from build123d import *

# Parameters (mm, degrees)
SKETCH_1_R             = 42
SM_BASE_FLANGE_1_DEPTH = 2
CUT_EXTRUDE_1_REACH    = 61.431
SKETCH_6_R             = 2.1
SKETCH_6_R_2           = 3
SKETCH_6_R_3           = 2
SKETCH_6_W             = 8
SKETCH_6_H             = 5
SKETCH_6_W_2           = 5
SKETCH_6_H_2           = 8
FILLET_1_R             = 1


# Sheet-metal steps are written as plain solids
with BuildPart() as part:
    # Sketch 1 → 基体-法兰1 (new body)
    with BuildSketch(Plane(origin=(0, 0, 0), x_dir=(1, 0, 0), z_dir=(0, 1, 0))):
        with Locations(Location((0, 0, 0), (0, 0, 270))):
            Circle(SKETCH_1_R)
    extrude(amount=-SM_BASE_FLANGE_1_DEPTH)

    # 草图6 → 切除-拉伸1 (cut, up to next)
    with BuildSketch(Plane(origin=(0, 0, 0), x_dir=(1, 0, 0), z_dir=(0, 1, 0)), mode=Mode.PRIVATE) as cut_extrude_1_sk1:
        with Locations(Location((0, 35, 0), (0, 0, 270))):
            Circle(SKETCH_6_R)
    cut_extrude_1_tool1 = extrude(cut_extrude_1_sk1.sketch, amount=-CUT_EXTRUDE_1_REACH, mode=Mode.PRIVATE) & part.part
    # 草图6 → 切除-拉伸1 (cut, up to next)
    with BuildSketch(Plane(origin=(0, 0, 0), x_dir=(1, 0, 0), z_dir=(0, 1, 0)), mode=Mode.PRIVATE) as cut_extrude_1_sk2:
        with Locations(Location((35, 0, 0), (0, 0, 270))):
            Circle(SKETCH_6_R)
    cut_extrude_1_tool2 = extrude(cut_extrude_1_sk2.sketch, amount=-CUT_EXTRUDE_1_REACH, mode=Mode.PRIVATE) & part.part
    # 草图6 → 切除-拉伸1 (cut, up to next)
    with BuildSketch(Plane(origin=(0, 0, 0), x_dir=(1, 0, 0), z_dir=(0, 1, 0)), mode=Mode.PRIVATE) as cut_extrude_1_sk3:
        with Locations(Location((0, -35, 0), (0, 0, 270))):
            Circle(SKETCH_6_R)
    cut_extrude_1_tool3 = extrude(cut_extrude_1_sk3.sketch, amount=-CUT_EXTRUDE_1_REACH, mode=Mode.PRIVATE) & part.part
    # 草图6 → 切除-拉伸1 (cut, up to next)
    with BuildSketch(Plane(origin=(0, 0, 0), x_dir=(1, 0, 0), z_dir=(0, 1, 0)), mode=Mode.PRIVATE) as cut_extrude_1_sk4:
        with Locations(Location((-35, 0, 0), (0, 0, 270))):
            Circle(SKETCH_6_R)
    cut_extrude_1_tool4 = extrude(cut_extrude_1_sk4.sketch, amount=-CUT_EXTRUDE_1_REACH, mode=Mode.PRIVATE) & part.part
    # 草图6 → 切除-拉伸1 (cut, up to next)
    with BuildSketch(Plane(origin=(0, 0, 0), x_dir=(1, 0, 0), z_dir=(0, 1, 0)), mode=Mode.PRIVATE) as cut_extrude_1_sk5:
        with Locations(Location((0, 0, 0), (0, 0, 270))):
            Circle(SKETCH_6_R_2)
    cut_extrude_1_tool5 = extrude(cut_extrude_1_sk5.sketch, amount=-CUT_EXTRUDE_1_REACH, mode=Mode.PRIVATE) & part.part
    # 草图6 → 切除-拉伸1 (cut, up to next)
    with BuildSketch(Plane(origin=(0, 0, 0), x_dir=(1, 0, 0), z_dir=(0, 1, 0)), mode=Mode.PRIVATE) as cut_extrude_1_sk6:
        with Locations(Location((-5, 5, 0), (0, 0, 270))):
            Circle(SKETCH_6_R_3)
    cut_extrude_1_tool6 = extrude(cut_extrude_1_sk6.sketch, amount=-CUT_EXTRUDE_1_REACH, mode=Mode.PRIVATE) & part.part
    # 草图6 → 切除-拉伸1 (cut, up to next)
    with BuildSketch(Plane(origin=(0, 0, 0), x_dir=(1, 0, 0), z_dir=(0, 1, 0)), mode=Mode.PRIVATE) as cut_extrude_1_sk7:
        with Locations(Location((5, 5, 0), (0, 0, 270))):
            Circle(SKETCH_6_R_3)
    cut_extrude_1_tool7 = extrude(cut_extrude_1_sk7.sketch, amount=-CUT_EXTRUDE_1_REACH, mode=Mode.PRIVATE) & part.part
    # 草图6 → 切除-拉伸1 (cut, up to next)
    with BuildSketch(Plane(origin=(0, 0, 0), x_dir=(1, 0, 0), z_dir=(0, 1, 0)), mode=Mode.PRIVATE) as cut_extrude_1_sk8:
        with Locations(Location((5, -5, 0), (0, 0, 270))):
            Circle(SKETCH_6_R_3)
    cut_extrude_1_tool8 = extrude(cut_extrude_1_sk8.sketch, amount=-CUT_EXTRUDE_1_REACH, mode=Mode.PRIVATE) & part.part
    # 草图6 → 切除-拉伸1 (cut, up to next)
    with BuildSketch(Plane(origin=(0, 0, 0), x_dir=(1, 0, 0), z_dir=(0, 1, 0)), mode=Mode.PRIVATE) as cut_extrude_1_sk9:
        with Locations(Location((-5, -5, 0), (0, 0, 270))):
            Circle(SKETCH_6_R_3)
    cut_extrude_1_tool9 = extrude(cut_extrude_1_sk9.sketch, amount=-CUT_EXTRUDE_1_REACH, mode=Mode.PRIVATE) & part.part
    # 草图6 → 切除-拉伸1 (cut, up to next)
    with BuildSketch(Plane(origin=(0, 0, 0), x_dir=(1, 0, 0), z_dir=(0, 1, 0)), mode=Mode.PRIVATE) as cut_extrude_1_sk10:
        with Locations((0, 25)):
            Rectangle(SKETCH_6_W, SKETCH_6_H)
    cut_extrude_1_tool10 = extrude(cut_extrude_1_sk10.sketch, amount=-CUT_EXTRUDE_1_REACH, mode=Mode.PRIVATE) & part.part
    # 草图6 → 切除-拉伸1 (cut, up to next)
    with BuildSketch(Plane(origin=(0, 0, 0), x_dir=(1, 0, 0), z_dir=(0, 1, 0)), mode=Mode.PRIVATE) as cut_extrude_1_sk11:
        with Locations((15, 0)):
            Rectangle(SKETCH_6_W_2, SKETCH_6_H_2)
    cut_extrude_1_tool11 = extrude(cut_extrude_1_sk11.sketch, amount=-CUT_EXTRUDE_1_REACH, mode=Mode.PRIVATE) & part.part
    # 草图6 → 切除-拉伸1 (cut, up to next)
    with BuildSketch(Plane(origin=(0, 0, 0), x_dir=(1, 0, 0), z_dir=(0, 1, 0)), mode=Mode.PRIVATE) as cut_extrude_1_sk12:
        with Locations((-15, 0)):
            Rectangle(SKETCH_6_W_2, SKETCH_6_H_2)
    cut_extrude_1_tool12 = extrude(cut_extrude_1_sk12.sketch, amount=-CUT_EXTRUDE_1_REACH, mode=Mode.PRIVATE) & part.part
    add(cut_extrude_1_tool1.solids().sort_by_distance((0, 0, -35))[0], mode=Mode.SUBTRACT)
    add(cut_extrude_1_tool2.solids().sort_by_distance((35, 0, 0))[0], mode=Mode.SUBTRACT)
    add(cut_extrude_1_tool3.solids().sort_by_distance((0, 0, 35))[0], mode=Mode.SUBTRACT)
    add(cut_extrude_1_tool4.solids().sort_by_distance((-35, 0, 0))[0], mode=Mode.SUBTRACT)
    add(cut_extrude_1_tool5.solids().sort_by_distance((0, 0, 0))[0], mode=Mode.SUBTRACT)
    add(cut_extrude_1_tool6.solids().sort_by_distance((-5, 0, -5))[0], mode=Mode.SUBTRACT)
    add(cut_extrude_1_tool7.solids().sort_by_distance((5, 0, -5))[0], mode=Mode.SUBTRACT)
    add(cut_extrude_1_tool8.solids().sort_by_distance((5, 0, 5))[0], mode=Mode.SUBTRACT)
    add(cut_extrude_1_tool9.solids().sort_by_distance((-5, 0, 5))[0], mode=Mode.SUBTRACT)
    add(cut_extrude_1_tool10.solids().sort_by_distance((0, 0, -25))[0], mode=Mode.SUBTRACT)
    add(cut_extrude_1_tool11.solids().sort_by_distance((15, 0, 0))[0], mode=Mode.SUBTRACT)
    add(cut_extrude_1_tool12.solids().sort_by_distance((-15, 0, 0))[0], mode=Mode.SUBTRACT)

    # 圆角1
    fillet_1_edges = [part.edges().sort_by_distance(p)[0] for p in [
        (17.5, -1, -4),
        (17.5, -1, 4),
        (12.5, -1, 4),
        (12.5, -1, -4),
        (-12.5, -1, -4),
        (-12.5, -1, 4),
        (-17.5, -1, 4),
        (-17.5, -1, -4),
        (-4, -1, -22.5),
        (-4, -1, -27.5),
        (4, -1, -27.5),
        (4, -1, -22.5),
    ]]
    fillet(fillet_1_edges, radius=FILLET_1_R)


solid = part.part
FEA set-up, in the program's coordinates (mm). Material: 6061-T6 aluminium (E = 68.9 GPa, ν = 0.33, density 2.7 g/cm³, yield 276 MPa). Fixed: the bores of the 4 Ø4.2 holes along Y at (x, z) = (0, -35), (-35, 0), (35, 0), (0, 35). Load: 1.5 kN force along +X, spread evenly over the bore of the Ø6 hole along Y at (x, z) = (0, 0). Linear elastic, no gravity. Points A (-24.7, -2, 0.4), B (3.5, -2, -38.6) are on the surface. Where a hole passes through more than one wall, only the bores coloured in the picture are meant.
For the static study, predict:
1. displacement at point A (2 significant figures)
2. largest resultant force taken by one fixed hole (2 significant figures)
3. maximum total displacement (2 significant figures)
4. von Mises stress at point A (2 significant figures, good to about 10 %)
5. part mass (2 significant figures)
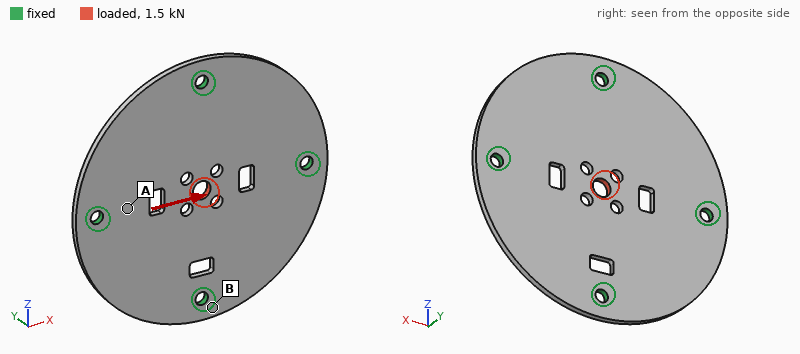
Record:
2.2 µm
460 N
14 µm
13 MPa
29 g
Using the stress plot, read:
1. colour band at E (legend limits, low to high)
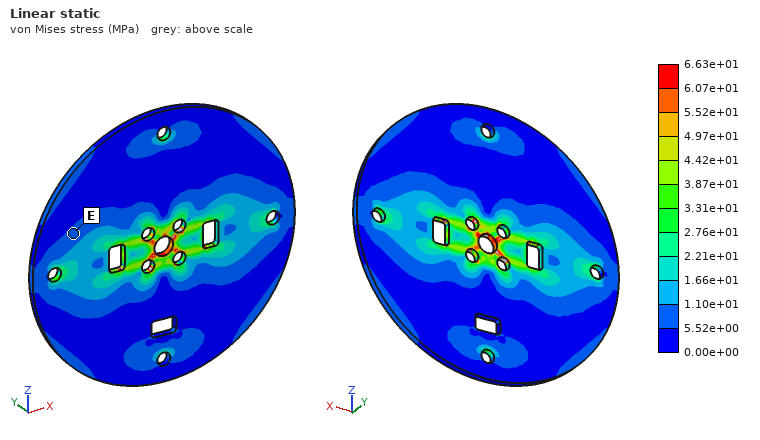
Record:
5.52e+00 to 1.10e+01 MPa
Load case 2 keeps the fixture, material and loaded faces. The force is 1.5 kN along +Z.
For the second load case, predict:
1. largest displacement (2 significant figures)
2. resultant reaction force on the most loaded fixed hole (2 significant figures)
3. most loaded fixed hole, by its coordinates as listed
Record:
13 µm
530 N
(0, 35)
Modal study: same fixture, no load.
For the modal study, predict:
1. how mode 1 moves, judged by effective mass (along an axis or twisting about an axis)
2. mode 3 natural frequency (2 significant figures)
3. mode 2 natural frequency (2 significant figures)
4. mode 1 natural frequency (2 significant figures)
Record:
along Y
3600 Hz
3500 Hz
3200 Hz
